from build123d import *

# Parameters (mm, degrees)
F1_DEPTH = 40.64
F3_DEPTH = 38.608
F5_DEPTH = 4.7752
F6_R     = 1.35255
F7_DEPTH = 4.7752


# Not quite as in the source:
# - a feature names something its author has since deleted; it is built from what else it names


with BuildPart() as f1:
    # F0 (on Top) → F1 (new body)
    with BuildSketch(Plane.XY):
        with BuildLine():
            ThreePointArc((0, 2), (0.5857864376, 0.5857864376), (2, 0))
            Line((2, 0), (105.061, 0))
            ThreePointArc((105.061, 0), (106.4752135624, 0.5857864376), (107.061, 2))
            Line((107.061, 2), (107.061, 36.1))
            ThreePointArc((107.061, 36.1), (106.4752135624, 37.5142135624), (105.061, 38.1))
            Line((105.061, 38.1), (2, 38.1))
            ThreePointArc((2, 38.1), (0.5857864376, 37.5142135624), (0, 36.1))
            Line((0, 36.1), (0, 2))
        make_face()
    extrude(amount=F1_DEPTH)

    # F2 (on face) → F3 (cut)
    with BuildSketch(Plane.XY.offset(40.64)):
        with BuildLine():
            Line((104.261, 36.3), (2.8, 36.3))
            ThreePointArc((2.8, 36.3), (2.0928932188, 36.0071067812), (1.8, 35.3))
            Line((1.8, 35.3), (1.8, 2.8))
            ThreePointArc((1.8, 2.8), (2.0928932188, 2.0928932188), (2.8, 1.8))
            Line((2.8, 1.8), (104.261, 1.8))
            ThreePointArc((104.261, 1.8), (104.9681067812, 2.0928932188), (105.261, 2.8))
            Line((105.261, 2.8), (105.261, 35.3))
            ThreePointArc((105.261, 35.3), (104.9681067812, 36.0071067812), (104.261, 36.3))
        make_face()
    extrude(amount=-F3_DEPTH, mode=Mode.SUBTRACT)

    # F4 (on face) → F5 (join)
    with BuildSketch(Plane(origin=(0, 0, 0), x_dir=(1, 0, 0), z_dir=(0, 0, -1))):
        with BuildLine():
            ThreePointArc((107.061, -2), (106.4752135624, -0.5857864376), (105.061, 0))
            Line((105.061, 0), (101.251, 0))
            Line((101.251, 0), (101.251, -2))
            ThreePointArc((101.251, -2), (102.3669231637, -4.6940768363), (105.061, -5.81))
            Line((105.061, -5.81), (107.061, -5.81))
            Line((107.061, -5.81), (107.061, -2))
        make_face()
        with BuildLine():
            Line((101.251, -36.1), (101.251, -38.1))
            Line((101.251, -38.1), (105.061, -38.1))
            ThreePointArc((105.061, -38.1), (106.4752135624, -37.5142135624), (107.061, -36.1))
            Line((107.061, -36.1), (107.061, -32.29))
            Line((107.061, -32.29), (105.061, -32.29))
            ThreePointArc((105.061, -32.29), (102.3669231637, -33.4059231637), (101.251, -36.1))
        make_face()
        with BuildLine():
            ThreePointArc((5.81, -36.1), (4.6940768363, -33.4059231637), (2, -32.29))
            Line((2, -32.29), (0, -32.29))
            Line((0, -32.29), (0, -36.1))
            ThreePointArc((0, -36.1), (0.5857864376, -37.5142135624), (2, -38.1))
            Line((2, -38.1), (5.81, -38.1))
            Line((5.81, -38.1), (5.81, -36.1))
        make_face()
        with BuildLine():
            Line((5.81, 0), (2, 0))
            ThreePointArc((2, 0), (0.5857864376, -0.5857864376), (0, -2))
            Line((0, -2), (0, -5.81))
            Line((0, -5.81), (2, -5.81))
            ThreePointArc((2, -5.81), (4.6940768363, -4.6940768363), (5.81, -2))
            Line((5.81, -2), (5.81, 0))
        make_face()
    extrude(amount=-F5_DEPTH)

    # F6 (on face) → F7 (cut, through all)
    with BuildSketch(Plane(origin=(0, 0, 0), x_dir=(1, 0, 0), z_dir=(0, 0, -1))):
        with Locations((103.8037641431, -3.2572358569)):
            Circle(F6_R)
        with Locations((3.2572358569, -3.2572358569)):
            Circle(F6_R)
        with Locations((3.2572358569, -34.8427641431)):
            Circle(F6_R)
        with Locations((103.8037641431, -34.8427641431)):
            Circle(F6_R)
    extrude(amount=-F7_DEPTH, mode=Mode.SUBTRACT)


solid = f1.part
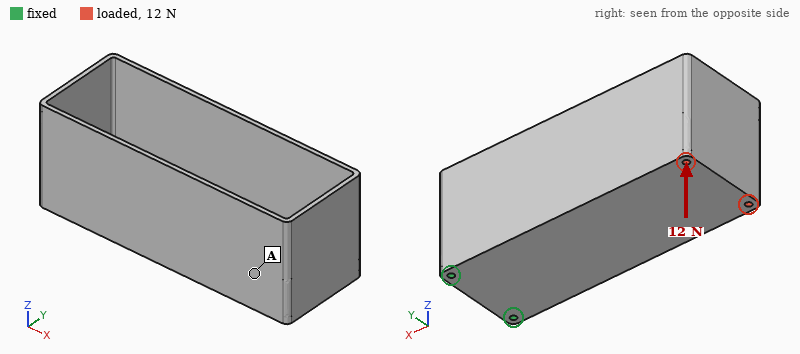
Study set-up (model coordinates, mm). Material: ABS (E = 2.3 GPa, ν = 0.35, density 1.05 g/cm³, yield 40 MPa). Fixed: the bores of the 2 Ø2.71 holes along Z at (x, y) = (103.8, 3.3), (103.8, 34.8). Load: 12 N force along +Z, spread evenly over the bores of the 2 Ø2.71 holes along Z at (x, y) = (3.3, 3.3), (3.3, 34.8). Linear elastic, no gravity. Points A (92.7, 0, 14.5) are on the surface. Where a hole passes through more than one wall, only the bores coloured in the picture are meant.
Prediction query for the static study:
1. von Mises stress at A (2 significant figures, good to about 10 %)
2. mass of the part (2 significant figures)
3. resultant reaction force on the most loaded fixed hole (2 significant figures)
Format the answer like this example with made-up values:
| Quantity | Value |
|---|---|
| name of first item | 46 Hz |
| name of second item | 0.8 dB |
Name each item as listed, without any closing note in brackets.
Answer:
| Quantity | Value |
|---|---|
| von Mises stress at A | 1.3 MPa |
| mass of the part | 29 g |
| resultant reaction force on the most loaded fixed hole | 6.4 N |
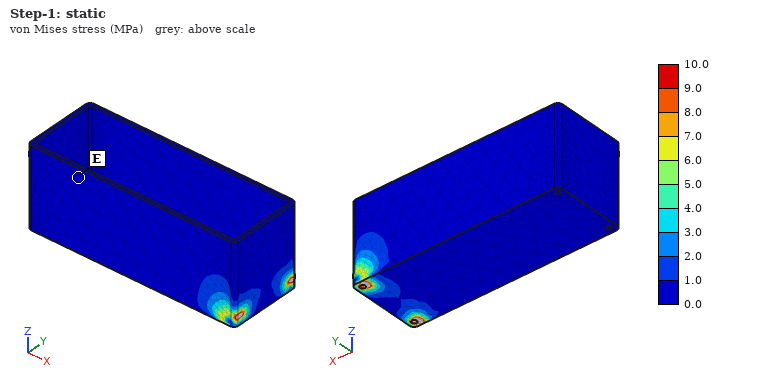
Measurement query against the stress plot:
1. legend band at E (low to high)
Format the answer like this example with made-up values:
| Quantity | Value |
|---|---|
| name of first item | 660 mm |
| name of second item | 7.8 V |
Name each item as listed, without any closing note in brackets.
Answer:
| Quantity | Value |
|---|---|
| legend band at E | 0.0 to 1.0 MPa |
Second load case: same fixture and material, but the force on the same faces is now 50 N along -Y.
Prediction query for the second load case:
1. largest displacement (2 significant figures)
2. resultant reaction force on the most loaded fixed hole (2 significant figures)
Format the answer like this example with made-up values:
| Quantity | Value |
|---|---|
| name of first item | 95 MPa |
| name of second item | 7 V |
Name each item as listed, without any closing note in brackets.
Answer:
| Quantity | Value |
|---|---|
| largest displacement | 1.4 mm |
| resultant reaction force on the most loaded fixed hole | 150 N |
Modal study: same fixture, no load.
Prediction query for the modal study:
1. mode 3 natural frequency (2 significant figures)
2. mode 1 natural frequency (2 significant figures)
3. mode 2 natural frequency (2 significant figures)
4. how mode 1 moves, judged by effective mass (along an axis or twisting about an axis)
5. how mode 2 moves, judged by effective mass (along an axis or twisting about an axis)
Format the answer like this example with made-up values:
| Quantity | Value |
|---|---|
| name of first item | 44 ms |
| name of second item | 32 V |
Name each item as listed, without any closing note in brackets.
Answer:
| Quantity | Value |
|---|---|
| mode 3 natural frequency | 350 Hz |
| mode 1 natural frequency | 140 Hz |
| mode 2 natural frequency | 150 Hz |
| how mode 1 moves, judged by effective mass | along Z |
| how mode 2 moves, judged by effective mass | along Y |
